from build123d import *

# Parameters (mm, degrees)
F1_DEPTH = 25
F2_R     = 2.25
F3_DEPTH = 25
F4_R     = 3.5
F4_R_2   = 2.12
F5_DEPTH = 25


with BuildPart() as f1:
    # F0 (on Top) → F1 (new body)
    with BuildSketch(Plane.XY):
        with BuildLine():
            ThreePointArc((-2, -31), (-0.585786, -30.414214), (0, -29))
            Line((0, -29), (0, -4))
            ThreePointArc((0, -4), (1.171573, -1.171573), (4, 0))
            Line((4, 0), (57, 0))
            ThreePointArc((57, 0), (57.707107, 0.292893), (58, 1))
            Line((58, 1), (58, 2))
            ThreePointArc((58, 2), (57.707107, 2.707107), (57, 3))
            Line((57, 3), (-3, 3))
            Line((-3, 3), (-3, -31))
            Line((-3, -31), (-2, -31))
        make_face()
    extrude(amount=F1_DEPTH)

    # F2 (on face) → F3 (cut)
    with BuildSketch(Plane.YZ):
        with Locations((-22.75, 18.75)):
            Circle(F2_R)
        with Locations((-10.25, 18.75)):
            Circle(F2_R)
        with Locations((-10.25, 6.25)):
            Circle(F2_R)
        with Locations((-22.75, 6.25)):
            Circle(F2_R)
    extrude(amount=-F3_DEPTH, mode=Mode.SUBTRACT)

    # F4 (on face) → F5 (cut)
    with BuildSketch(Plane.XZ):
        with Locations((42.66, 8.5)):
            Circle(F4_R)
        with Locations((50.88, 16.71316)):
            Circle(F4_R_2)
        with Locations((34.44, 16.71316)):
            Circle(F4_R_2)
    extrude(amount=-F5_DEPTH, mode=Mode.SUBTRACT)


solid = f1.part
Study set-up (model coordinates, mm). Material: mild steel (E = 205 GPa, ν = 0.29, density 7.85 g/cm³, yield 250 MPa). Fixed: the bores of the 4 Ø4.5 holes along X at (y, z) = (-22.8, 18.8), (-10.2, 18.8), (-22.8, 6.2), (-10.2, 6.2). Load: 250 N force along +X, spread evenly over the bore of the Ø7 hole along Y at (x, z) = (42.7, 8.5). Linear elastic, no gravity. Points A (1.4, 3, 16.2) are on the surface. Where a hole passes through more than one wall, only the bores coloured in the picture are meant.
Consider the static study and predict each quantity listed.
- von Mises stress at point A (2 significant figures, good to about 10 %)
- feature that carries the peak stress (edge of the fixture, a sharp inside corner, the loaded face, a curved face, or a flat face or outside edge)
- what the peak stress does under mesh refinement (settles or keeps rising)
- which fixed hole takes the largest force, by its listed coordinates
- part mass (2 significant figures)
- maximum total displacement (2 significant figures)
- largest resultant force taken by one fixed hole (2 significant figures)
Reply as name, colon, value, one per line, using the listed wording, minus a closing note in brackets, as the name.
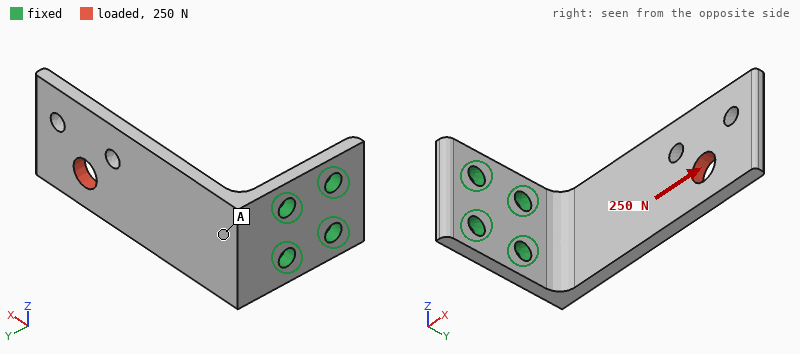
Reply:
von Mises stress at point A: 8.3 MPa
feature that carries the peak stress: edge of the fixture
what the peak stress does under mesh refinement: keeps rising
which fixed hole takes the largest force, by its listed coordinates: (-10.2, 6.2)
part mass: 52 g
maximum total displacement: 69 µm
largest resultant force taken by one fixed hole: 200 N
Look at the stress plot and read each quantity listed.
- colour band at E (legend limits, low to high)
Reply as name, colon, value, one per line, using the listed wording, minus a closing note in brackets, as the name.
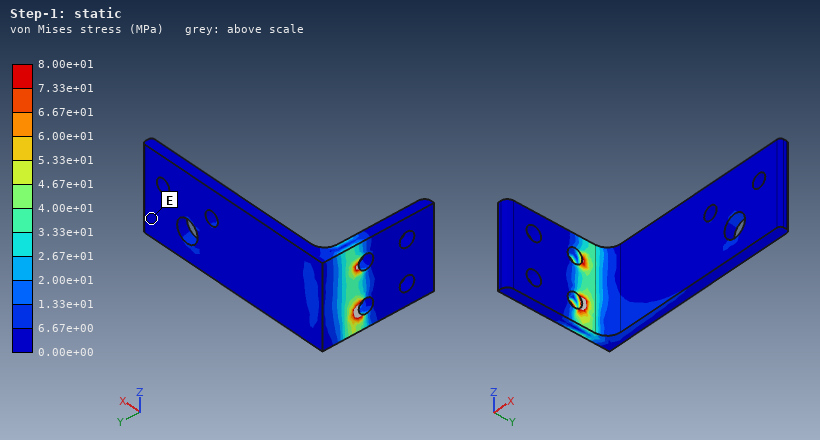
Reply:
colour band at E: 0.00e+00 to 6.67e+00 MPa
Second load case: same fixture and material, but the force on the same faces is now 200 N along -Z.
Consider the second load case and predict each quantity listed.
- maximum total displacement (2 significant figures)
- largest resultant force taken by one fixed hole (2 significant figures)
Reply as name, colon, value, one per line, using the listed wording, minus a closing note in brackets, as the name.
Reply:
maximum total displacement: 0.11 mm
largest resultant force taken by one fixed hole: 570 N
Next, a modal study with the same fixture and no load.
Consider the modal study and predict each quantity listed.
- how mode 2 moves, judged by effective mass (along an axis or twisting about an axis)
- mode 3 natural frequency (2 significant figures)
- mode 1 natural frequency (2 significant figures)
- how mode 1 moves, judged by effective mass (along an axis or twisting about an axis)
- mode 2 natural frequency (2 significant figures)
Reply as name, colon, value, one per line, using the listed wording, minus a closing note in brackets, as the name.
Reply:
how mode 2 moves, judged by effective mass: along Z
mode 3 natural frequency: 3500 Hz
mode 1 natural frequency: 630 Hz
how mode 1 moves, judged by effective mass: along Y
mode 2 natural frequency: 1800 Hz
